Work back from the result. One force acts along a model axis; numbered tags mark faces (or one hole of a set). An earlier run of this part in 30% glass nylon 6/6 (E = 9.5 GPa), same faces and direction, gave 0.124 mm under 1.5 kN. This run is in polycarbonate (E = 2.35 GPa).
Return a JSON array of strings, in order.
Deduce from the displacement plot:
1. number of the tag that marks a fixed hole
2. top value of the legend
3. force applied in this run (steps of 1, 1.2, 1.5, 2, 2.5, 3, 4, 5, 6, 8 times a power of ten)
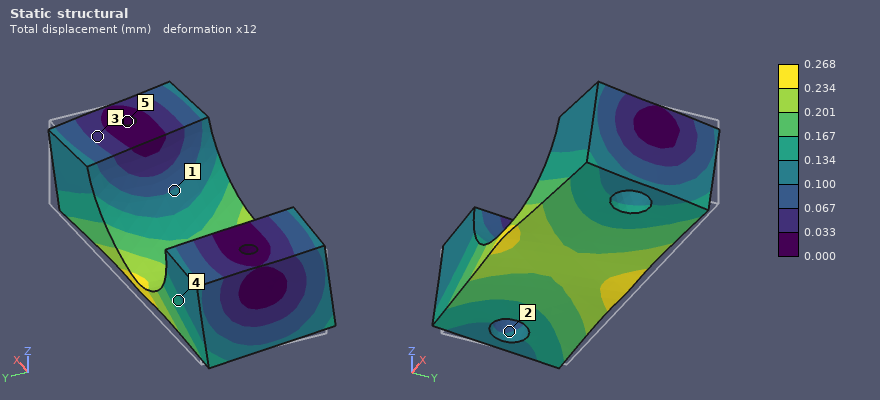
["5", "0.268 mm", "800 N"]
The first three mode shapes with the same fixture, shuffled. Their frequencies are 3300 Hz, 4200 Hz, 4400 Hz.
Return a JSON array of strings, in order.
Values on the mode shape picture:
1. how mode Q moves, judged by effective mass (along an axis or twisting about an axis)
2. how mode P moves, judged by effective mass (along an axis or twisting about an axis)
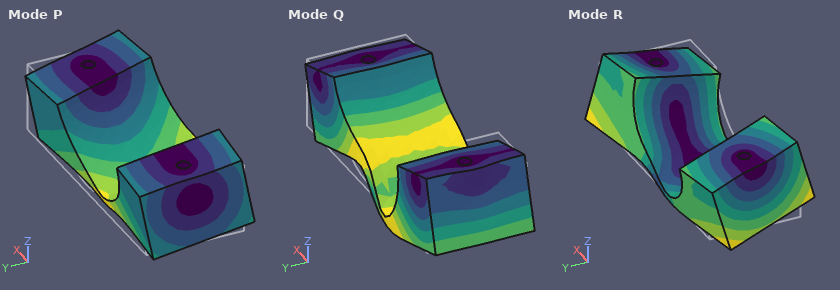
["along X", "along Y"]
